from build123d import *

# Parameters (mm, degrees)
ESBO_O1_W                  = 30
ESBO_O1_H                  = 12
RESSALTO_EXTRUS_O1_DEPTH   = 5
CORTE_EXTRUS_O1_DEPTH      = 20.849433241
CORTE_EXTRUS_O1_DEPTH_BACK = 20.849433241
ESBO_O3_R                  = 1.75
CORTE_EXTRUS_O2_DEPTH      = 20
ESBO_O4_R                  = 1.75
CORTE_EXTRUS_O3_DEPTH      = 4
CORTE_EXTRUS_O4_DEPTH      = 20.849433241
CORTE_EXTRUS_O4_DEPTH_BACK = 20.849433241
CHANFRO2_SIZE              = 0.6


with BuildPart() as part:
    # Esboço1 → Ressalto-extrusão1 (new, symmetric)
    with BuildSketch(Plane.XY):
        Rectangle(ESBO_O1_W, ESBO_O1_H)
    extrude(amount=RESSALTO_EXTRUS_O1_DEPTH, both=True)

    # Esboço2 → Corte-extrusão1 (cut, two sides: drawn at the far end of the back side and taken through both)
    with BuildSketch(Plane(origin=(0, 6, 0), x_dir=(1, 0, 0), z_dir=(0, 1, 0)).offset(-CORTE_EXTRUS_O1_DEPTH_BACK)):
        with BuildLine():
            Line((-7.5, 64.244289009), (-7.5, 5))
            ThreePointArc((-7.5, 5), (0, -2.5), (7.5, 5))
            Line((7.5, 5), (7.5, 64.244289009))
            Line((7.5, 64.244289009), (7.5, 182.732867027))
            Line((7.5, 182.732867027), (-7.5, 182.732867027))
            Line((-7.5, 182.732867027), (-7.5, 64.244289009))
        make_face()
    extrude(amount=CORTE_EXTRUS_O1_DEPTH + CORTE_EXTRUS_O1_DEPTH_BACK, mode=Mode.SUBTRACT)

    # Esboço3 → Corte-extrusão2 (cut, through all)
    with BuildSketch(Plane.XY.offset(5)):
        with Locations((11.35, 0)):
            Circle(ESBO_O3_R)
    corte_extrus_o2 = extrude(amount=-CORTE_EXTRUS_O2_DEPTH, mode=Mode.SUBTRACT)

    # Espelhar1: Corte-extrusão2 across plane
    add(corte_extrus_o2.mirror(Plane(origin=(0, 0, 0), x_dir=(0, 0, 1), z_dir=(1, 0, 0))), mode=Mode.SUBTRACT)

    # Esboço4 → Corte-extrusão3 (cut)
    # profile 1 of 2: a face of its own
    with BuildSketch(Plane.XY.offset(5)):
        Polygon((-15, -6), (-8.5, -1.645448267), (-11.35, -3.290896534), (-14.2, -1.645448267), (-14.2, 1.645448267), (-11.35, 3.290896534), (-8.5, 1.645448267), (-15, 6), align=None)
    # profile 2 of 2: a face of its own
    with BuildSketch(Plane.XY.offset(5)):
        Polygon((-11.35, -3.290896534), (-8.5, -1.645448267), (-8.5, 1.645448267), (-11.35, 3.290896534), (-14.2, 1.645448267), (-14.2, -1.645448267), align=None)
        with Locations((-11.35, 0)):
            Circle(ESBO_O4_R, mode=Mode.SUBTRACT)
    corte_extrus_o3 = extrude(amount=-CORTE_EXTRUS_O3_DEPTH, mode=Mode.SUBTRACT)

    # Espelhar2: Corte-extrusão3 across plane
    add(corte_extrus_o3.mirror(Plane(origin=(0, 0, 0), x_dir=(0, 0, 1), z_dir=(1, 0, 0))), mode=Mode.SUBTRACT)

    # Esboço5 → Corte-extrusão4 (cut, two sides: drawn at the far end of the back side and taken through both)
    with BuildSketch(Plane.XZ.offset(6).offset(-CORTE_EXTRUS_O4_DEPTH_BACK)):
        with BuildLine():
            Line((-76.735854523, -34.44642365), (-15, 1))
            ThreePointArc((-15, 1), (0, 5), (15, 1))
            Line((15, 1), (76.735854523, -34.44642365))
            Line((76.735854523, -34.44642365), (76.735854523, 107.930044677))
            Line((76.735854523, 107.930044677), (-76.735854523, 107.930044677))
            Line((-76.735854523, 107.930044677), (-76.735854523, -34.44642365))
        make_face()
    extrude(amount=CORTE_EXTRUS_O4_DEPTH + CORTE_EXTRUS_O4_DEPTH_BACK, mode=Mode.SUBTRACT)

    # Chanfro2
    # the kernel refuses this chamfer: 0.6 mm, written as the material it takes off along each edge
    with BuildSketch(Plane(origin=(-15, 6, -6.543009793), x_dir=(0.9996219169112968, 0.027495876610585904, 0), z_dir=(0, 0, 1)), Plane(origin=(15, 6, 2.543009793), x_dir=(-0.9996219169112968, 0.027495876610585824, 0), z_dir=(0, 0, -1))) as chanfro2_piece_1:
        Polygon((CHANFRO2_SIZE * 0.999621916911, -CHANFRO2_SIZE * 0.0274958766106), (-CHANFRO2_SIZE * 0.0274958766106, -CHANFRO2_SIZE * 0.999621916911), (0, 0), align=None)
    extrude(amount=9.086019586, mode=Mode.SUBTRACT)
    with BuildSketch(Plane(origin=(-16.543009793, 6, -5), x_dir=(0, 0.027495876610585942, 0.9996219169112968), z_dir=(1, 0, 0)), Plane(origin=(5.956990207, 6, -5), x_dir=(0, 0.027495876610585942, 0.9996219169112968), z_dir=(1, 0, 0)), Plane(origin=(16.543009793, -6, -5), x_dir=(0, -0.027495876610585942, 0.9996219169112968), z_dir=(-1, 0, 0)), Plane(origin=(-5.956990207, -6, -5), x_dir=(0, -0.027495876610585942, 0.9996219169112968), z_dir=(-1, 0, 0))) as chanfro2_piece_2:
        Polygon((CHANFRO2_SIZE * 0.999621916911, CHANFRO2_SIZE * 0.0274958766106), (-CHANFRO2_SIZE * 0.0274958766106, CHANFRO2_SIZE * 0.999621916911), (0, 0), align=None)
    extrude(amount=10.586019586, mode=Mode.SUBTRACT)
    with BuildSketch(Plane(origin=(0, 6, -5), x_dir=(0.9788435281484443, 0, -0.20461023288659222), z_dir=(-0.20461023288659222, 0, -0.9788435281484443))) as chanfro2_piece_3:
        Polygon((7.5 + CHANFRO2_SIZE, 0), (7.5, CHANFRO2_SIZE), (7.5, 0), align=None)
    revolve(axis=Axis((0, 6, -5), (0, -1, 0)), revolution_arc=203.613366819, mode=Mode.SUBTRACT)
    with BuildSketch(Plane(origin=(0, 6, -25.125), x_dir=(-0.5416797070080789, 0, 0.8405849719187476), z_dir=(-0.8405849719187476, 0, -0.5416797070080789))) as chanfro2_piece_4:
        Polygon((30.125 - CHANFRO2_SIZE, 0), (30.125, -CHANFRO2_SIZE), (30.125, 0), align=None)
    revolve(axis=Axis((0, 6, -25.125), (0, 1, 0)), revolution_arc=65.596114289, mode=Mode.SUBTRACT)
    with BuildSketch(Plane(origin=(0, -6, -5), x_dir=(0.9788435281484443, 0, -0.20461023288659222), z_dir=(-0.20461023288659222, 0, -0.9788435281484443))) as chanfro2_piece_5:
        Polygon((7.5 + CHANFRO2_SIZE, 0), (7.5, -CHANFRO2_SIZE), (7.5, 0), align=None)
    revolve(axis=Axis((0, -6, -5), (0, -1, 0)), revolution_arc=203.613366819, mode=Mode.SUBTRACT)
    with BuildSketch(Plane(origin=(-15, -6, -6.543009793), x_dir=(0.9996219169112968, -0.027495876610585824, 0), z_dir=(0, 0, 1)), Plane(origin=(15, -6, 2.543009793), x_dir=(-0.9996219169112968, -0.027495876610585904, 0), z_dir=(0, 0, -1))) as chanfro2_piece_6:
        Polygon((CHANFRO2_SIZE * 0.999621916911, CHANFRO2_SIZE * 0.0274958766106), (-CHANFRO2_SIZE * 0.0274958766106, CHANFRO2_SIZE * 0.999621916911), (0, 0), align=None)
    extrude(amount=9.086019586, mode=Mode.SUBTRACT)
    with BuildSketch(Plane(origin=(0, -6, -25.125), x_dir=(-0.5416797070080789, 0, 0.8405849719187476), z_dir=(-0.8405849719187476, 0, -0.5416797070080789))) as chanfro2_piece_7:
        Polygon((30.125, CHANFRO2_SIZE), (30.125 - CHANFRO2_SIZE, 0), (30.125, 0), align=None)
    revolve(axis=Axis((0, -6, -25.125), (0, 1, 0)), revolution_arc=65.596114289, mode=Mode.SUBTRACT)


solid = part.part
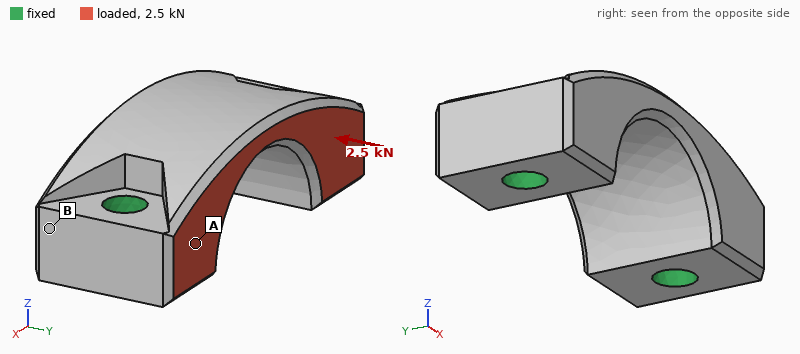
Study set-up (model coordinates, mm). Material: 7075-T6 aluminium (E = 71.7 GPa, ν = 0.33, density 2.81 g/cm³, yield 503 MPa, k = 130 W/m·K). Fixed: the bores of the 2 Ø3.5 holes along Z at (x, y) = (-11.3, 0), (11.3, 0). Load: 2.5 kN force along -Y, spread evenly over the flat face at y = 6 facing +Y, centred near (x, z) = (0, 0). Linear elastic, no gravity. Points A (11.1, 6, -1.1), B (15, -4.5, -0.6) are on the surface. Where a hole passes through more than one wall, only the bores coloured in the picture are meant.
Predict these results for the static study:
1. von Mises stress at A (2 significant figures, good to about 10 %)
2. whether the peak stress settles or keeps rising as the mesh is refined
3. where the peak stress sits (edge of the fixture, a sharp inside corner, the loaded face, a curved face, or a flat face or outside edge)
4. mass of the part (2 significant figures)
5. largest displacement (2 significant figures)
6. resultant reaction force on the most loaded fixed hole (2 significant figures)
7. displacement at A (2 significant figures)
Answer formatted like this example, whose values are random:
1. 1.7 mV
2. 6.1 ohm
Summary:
1. 29 MPa
2. keeps rising
3. edge of the fixture
4. 5.1 g
5. 10 µm
6. 1.3 kN
7. 3.2 µm
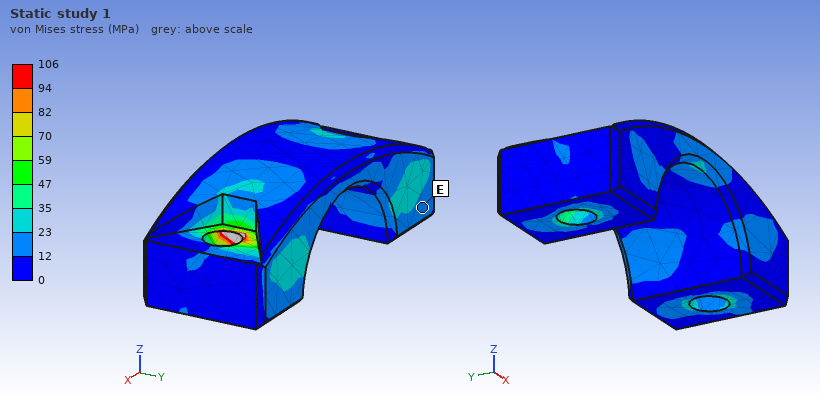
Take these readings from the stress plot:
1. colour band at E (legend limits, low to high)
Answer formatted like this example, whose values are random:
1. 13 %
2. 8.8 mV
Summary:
1. 12 to 23 MPa
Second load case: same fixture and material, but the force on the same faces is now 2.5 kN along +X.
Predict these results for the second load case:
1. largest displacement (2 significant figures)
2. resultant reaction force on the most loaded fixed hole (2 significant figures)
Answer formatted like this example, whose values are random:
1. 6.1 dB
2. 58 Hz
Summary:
1. 9.4 µm
2. 1.3 kN
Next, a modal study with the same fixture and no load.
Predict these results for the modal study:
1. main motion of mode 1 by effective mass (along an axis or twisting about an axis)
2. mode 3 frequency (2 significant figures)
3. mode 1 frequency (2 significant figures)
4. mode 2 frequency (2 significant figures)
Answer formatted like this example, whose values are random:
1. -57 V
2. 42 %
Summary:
1. along Y
2. 60 kHz
3. 39 kHz
4. 59 kHz
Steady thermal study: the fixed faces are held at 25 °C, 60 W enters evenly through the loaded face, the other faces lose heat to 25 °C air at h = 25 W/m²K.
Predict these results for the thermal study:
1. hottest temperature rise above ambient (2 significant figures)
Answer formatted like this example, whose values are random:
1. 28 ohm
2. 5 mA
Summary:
1. 25 K
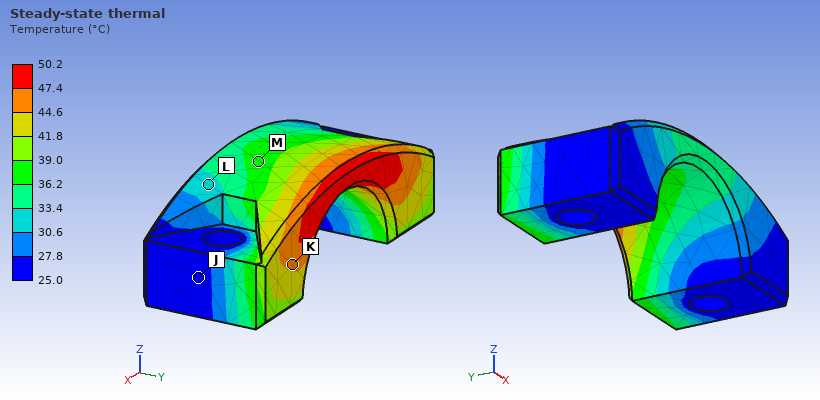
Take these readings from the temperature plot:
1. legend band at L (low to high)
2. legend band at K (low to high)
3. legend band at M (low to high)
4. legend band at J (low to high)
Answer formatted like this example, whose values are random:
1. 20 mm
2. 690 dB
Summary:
1. 30.6 to 33.4 °C
2. 44.6 to 47.4 °C
3. 36.2 to 39.0 °C
4. 25.0 to 27.8 °C
